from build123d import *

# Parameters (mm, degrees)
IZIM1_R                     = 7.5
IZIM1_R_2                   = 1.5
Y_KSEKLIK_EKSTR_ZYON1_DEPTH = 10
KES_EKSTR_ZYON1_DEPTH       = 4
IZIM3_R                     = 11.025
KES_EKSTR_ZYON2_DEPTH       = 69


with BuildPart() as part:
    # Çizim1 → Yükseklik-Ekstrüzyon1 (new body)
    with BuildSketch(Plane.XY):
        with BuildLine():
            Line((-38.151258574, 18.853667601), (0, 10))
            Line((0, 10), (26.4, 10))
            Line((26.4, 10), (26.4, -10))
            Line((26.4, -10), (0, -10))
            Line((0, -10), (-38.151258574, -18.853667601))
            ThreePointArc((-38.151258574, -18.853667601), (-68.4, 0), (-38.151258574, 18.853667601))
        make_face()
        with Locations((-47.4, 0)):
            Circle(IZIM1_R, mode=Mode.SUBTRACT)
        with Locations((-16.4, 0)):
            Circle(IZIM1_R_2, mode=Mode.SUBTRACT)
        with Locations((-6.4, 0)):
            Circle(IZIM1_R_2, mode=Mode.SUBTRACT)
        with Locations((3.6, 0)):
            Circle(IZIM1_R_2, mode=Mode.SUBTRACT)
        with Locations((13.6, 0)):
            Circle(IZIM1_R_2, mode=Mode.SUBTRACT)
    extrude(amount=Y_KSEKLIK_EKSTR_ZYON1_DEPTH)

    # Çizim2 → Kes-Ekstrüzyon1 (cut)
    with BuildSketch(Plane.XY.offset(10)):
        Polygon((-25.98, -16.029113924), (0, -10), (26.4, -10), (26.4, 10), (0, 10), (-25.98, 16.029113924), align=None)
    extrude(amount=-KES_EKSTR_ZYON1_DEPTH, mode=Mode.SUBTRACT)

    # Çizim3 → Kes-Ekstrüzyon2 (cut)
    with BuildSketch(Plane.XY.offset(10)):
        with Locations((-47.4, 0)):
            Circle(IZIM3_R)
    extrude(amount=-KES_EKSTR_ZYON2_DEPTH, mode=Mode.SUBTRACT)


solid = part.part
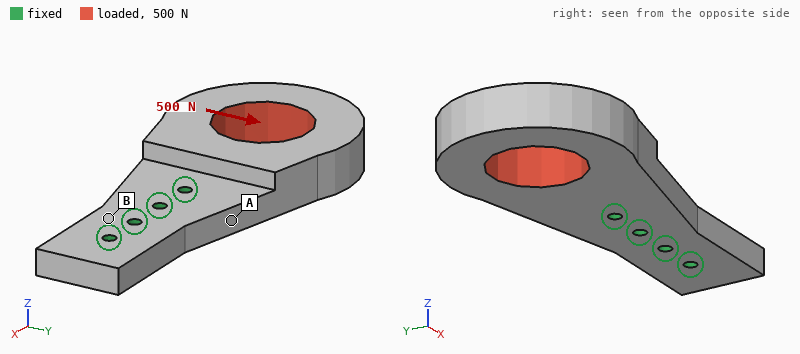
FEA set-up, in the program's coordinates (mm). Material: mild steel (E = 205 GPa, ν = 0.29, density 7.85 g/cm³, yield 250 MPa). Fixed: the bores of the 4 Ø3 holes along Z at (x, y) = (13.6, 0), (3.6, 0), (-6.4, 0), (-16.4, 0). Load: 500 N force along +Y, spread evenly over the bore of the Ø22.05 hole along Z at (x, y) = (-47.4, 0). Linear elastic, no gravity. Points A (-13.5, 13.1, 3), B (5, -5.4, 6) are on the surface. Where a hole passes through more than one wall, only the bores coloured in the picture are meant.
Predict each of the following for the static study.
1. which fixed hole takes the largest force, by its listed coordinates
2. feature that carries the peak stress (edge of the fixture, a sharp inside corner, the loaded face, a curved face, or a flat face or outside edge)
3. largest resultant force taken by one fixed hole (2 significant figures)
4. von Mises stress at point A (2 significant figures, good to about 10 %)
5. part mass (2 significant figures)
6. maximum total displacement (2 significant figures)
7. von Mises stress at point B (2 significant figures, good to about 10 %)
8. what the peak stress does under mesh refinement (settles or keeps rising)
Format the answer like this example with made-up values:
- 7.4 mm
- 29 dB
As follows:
- (-16.4, 0)
- edge of the fixture
- 1.3 kN
- 21 MPa
- 140 g
- 13 µm
- 3.5 MPa
- keeps rising
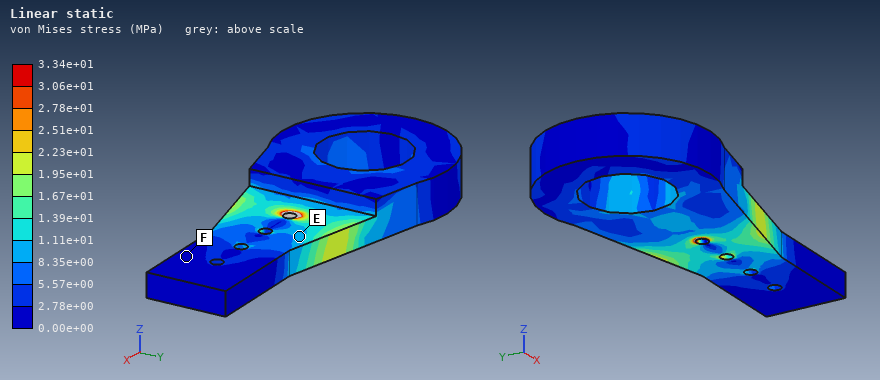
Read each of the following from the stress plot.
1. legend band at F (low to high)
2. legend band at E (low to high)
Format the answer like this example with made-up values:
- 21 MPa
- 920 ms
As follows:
- 0.00e+00 to 2.78e+00 MPa
- 8.35e+00 to 1.11e+01 MPa
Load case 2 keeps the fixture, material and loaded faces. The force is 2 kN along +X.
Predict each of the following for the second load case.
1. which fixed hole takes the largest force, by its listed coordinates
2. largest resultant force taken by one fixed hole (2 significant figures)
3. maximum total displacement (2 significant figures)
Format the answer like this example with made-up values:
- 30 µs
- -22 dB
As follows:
- (-16.4, 0)
- 1.2 kN
- 24 µm
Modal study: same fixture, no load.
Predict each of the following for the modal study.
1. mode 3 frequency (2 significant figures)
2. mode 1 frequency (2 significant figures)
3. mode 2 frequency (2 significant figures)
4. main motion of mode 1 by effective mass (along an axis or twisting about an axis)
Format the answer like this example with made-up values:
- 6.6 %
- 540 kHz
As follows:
- 4100 Hz
- 1600 Hz
- 3900 Hz
- along Z
